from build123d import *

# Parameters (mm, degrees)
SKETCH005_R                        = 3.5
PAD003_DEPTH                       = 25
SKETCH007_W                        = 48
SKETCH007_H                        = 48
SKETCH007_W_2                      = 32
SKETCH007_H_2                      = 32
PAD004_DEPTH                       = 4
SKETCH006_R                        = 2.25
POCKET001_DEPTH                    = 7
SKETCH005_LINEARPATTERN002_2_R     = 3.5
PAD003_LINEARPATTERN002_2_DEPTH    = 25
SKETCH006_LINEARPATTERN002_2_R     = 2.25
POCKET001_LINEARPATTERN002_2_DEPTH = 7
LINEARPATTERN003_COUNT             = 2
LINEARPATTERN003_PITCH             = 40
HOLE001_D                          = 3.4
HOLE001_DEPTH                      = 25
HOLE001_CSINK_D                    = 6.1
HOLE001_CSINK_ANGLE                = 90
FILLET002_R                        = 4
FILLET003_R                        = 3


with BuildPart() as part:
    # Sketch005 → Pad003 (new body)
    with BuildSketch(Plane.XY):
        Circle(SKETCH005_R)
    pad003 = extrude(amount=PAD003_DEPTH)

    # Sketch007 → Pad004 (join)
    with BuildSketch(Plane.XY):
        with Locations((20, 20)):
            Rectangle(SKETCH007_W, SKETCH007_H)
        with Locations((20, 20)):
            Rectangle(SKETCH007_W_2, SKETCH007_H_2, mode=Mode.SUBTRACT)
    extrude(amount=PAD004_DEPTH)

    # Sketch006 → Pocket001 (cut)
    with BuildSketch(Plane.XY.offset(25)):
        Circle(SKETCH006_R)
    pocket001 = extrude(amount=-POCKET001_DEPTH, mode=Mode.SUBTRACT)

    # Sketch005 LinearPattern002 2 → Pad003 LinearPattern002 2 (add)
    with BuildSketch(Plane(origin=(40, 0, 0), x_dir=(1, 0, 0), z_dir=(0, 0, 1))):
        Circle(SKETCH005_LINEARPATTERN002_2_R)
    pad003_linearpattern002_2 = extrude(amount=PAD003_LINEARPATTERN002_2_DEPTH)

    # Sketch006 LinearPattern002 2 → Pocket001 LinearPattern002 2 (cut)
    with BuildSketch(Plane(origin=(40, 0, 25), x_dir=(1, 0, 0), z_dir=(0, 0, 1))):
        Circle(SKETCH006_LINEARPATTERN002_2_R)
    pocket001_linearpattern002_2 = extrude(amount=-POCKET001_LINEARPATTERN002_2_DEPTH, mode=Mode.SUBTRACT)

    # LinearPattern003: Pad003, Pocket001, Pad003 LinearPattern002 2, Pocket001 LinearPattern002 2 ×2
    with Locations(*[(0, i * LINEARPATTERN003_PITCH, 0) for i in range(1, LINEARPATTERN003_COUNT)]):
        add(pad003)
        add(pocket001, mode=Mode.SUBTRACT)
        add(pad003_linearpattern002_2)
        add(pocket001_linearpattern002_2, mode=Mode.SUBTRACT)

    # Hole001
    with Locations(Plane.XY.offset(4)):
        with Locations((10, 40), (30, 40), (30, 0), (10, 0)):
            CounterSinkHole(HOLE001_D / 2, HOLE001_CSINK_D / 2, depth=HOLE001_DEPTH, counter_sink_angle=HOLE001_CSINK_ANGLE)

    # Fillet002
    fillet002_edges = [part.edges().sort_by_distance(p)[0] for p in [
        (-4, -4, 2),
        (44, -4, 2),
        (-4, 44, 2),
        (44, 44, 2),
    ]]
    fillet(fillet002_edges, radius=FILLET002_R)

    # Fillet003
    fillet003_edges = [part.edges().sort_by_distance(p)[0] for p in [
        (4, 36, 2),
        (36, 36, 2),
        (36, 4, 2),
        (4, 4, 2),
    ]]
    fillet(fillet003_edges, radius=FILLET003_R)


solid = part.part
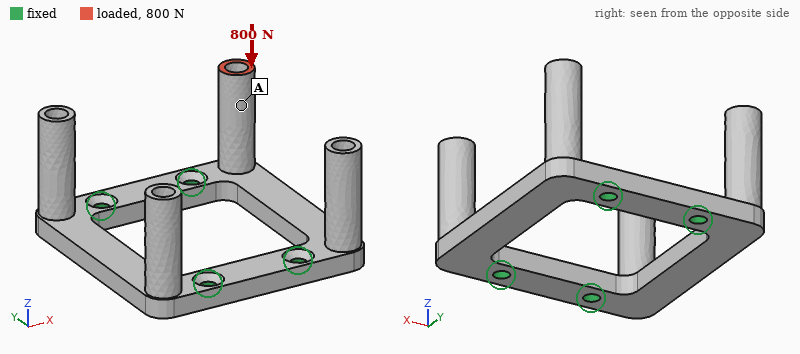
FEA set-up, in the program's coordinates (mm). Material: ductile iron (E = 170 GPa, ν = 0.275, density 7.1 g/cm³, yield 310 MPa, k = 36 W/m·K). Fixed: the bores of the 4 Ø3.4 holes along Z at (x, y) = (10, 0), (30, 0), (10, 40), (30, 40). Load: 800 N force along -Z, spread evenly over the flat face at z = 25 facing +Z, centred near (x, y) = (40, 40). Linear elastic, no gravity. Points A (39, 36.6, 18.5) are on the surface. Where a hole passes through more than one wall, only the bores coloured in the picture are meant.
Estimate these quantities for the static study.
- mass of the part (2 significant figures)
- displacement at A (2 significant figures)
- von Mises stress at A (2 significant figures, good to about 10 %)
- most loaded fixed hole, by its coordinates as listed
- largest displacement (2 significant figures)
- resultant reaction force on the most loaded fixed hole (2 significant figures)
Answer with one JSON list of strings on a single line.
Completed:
["55 g", "0.089 mm", "30 MPa", "(30, 40)", "0.13 mm", "830 N"]
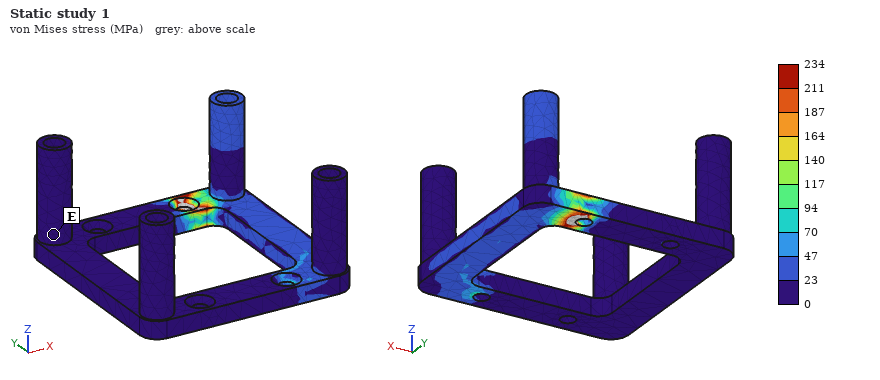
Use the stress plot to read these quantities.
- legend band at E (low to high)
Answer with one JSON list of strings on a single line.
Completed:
["0 to 23 MPa"]
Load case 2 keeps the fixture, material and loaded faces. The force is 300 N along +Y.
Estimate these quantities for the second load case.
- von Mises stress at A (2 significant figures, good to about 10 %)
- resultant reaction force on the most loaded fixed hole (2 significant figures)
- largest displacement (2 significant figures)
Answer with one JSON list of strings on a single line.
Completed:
["68 MPa", "200 N", "0.16 mm"]
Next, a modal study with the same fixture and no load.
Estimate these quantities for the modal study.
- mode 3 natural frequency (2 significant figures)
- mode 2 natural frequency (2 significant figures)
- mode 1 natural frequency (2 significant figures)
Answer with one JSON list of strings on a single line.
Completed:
["4800 Hz", "3800 Hz", "3800 Hz"]
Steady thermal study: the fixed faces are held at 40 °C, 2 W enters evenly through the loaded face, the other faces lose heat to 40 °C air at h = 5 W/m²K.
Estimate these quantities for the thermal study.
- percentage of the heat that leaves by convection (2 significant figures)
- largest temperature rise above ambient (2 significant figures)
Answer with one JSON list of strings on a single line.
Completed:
["6.4 %", "49 K"]
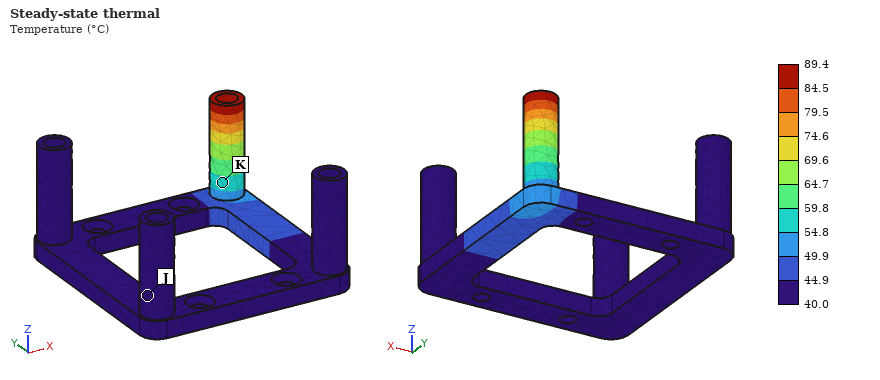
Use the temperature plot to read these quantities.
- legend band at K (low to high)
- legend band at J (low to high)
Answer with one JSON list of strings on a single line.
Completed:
["54.8 to 59.8 °C", "40.0 to 44.9 °C"]
